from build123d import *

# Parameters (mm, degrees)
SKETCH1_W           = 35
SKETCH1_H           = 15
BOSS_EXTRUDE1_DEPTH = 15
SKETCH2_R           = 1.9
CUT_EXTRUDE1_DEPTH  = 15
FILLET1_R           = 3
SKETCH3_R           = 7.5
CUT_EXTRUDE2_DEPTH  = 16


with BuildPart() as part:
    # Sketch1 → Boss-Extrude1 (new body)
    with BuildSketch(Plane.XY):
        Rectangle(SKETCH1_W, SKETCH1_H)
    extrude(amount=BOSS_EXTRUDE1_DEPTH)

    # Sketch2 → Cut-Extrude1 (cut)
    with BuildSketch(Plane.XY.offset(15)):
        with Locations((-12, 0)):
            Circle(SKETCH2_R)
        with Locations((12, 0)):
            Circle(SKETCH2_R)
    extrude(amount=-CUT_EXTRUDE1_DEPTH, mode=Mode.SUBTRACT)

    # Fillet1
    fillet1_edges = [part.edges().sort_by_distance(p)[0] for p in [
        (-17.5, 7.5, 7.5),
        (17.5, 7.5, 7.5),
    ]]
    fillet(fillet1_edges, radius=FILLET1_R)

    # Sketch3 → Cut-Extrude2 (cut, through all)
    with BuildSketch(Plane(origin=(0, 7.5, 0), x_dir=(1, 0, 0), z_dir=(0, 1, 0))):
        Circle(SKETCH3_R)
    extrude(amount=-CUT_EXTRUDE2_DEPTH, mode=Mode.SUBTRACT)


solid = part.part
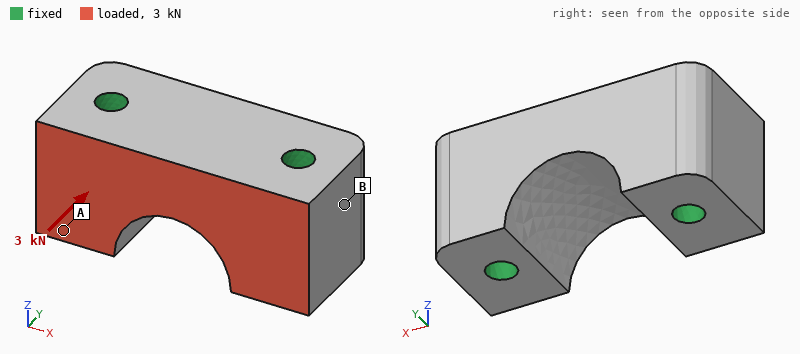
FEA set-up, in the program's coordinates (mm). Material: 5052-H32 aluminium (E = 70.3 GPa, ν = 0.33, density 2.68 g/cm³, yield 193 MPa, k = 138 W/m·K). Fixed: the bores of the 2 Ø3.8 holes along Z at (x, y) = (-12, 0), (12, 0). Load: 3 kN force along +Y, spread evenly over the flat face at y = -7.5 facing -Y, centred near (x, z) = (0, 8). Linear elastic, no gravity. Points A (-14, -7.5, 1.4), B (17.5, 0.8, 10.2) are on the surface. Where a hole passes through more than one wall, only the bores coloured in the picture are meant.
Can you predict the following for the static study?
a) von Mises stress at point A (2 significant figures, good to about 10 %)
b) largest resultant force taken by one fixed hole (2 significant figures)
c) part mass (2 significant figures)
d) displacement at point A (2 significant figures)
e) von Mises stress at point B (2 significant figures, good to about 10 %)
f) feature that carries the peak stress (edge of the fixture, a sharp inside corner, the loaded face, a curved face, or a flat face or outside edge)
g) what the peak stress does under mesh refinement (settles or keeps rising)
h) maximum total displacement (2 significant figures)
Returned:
8.1 MPa
1.5 kN
16 g
0.70 µm
4.0 MPa
edge of the fixture
keeps rising
2.5 µm
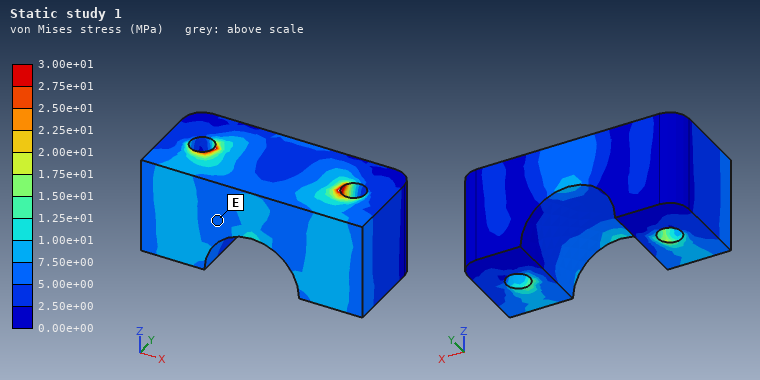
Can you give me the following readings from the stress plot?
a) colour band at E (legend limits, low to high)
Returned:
5.00e+00 to 7.50e+00 MPa
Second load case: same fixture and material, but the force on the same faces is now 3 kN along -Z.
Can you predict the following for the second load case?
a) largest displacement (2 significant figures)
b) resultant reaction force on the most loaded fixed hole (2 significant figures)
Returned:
6.7 µm
1.5 kN
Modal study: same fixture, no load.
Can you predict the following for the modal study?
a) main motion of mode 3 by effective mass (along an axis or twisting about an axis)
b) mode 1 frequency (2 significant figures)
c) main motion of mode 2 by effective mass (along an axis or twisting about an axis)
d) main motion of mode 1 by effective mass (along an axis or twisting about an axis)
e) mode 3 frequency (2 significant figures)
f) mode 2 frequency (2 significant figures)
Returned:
twisting about X
50 kHz
along Z
along Y
71 kHz
60 kHz
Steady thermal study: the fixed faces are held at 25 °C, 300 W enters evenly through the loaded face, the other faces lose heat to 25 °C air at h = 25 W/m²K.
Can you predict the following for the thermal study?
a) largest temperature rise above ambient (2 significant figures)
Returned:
50 K
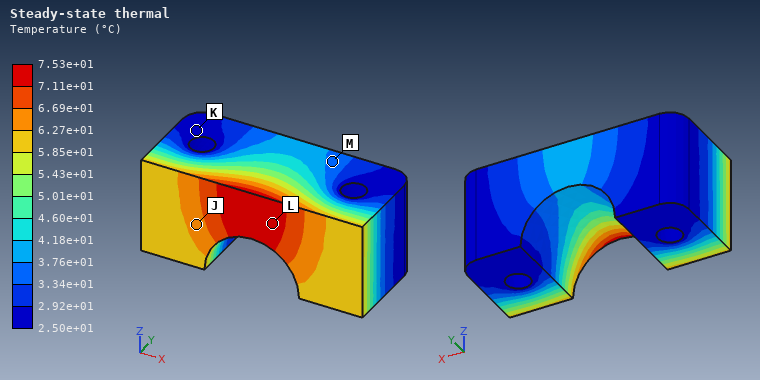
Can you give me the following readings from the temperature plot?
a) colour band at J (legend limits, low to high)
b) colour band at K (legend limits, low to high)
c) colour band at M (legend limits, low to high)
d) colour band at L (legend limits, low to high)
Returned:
6.27e+01 to 6.69e+01 °C
2.50e+01 to 2.92e+01 °C
3.34e+01 to 3.76e+01 °C
7.11e+01 to 7.53e+01 °C
